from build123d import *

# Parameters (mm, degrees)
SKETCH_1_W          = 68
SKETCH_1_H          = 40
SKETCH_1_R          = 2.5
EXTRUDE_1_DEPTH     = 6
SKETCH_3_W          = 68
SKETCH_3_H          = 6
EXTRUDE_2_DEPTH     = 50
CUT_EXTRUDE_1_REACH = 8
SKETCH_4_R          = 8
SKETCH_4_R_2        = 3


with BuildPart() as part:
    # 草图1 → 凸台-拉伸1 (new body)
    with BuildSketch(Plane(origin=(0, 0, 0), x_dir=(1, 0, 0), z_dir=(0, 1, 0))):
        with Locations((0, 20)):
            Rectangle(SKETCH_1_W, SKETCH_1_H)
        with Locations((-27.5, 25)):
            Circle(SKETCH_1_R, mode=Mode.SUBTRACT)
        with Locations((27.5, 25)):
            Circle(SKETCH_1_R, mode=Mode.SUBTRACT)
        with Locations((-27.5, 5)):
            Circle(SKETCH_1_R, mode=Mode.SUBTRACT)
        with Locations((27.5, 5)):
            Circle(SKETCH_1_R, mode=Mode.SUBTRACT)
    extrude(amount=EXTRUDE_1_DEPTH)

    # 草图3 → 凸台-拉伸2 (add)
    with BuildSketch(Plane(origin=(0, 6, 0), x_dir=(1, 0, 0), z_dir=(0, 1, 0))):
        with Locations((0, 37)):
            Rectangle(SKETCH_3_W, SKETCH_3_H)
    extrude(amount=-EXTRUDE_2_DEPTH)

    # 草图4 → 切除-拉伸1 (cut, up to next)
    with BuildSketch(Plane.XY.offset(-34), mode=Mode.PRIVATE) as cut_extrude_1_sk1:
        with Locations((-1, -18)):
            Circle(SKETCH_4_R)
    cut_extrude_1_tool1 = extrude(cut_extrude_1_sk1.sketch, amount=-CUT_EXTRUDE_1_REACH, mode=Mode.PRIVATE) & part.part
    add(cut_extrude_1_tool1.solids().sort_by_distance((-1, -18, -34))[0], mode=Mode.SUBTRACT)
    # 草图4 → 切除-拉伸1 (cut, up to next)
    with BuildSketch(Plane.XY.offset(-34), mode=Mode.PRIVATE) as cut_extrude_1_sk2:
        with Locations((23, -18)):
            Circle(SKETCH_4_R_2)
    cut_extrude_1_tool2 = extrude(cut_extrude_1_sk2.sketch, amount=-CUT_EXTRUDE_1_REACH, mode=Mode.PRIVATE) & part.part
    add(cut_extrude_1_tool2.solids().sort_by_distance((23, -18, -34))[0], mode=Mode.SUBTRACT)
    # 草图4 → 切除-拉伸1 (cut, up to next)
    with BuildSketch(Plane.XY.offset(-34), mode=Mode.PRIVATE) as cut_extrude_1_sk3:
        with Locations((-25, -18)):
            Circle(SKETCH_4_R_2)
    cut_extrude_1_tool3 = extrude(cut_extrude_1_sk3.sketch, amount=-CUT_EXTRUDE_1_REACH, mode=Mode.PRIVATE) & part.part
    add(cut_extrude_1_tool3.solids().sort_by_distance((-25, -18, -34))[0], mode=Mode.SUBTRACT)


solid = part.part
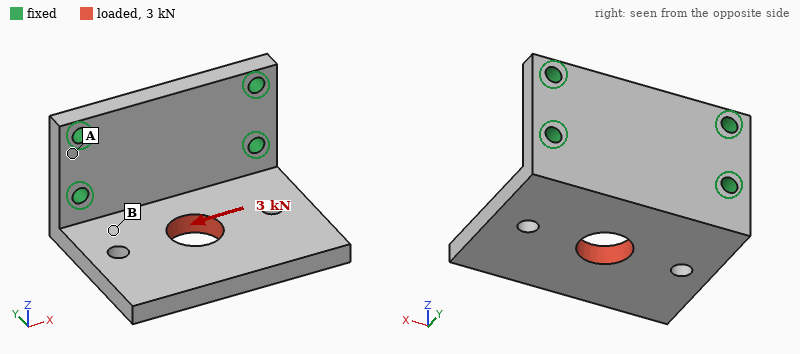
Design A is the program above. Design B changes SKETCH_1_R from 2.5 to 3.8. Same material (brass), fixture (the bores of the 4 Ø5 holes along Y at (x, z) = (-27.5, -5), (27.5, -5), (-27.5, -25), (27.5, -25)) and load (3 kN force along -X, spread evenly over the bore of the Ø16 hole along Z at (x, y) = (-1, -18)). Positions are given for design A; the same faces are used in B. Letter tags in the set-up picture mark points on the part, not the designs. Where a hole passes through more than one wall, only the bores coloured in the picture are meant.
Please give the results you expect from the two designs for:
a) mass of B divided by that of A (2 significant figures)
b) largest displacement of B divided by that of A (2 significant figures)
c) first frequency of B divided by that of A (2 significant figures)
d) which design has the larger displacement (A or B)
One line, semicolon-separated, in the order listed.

0.98; 0.79; 1.0; A
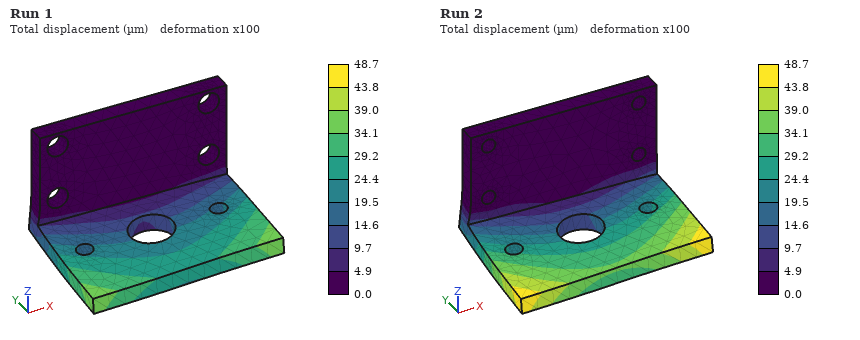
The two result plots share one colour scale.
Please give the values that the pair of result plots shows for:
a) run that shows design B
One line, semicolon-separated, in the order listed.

Run 1
